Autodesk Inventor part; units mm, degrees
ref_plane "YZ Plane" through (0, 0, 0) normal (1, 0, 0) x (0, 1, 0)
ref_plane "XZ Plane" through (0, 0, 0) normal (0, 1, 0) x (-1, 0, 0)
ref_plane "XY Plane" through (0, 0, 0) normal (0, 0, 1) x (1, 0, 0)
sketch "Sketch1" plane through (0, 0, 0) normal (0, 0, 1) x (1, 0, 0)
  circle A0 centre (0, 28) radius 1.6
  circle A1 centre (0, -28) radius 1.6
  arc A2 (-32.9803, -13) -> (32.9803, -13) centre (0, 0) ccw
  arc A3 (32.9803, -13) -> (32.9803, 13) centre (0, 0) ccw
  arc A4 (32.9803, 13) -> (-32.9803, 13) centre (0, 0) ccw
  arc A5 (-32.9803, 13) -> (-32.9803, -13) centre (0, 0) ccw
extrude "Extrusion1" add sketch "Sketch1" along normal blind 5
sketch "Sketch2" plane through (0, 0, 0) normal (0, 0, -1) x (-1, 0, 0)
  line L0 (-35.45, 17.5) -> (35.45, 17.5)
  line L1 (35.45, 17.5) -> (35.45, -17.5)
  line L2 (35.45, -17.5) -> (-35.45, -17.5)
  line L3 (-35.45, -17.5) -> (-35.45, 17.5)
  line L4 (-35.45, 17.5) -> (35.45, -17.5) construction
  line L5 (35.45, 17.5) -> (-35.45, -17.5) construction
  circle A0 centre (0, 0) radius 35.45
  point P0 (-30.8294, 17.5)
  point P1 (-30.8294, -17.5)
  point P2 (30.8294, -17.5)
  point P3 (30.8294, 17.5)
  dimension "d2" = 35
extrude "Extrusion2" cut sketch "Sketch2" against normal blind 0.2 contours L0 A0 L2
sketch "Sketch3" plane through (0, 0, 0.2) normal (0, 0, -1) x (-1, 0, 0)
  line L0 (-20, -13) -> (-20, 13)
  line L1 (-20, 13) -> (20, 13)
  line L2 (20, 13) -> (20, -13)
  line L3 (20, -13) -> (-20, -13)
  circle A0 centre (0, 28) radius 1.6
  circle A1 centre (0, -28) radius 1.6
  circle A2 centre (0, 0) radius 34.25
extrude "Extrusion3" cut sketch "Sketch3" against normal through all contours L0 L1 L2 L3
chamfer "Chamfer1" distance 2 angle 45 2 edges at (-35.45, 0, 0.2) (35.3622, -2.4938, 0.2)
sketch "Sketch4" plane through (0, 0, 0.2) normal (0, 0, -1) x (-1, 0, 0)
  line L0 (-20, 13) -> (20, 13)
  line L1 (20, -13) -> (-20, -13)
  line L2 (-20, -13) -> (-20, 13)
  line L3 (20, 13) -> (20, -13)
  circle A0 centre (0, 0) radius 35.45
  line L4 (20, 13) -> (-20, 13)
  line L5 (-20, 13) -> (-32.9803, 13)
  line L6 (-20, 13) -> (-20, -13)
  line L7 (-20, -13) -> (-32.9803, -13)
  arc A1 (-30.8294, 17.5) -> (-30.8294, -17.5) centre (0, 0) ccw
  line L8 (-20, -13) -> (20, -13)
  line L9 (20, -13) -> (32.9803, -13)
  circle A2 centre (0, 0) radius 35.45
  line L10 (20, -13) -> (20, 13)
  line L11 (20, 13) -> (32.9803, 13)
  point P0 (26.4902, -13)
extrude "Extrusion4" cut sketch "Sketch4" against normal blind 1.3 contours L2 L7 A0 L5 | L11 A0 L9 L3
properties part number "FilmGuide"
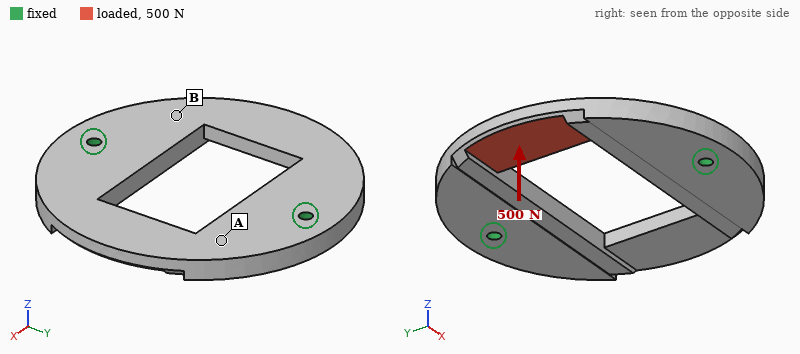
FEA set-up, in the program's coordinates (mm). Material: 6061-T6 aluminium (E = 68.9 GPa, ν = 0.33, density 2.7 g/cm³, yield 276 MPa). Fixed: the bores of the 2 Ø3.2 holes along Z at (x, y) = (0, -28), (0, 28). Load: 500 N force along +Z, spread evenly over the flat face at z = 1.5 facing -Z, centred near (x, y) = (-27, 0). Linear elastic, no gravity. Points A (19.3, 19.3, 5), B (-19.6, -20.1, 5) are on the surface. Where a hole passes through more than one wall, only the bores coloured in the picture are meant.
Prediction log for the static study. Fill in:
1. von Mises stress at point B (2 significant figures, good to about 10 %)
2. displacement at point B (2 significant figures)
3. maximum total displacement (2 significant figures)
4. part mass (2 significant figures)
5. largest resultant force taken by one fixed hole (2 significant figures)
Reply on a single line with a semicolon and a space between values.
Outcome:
39 MPa; 0.11 mm; 0.31 mm; 36 g; 270 N
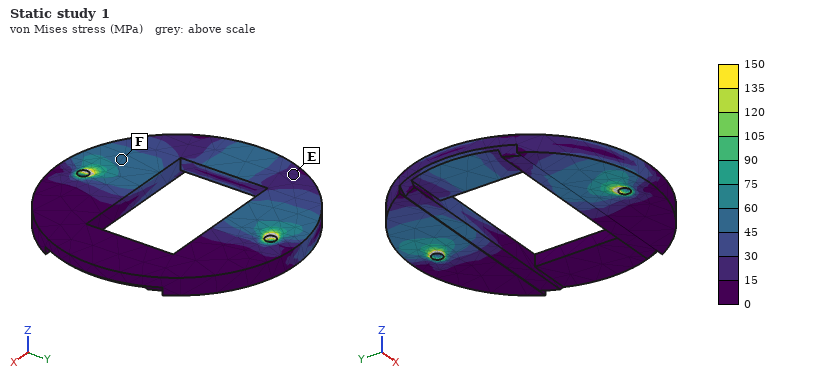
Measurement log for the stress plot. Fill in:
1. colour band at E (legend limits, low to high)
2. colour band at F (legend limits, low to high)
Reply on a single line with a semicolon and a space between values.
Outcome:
15 to 30 MPa; 45 to 60 MPa
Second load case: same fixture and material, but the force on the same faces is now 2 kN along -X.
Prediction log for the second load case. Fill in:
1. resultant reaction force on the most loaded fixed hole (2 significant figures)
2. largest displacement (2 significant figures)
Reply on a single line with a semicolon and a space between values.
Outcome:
1.1 kN; 78 µm
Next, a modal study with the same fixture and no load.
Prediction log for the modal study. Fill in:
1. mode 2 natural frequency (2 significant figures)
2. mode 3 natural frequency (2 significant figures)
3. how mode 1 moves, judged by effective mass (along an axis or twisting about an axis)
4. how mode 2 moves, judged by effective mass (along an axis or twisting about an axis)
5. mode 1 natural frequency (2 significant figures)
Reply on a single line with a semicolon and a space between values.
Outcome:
3400 Hz; 6000 Hz; twisting about Y; along Z; 2800 Hz
